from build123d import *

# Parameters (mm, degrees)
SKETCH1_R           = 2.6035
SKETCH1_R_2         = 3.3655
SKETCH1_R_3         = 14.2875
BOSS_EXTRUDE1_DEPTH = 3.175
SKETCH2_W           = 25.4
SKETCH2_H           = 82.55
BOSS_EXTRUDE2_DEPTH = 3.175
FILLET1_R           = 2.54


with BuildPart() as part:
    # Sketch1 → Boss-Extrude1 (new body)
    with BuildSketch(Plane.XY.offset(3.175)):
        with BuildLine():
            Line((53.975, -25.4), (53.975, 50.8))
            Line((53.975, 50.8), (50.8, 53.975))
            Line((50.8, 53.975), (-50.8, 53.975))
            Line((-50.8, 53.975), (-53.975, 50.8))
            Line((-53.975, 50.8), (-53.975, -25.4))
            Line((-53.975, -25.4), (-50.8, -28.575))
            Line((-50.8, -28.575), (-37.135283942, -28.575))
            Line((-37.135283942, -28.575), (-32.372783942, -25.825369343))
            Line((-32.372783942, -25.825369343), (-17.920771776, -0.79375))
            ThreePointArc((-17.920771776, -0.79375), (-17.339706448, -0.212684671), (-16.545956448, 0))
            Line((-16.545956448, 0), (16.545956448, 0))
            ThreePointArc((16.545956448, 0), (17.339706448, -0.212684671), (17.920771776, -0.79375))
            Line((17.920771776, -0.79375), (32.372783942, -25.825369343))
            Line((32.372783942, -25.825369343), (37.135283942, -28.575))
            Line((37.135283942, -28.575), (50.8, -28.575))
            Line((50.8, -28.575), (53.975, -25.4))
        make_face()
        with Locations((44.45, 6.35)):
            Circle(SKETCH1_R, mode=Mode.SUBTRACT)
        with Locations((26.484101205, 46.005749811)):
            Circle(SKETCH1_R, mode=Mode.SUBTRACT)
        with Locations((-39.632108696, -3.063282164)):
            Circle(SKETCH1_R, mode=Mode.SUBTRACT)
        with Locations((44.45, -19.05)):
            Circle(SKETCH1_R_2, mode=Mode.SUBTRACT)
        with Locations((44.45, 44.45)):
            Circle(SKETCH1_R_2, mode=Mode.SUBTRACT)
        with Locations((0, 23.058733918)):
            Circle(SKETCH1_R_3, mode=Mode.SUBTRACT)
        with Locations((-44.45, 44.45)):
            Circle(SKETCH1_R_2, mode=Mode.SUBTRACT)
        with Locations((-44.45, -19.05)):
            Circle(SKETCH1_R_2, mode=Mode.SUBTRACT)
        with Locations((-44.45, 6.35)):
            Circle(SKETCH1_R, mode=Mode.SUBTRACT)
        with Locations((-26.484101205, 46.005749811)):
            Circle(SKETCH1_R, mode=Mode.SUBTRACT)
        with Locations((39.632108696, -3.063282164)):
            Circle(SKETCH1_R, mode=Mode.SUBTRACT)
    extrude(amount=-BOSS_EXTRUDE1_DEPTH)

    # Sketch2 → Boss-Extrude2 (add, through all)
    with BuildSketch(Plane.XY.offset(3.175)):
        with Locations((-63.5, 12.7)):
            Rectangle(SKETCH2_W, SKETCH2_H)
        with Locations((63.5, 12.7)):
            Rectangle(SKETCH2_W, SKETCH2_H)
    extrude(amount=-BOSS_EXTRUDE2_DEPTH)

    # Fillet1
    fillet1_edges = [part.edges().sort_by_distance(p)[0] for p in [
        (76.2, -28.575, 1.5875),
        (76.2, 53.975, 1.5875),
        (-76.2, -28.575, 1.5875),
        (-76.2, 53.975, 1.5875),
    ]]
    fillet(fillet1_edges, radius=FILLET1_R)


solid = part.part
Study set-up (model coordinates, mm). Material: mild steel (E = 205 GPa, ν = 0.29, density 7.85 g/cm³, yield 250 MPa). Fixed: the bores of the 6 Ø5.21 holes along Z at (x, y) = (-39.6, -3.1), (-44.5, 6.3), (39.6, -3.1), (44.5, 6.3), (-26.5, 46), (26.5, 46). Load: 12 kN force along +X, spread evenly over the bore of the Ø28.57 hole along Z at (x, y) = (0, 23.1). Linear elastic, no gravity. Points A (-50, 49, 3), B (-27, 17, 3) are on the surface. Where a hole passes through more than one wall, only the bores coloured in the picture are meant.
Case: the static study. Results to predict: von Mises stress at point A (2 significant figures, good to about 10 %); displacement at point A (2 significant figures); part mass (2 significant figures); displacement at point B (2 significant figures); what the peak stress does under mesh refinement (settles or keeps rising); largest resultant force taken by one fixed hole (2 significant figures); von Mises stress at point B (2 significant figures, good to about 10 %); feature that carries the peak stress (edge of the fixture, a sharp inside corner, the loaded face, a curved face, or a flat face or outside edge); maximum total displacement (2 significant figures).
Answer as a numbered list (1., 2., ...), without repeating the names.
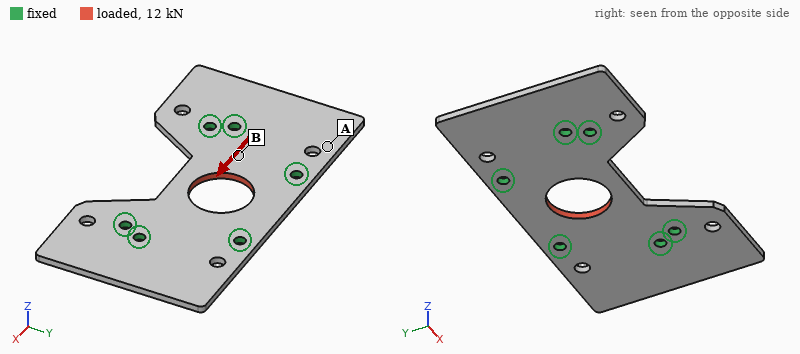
1. 11 MPa
2. 1.8 µm
3. 250 g
4. 4.2 µm
5. keeps rising
6. 3.0 kN
7. 34 MPa
8. edge of the fixture
9. 7.7 µm
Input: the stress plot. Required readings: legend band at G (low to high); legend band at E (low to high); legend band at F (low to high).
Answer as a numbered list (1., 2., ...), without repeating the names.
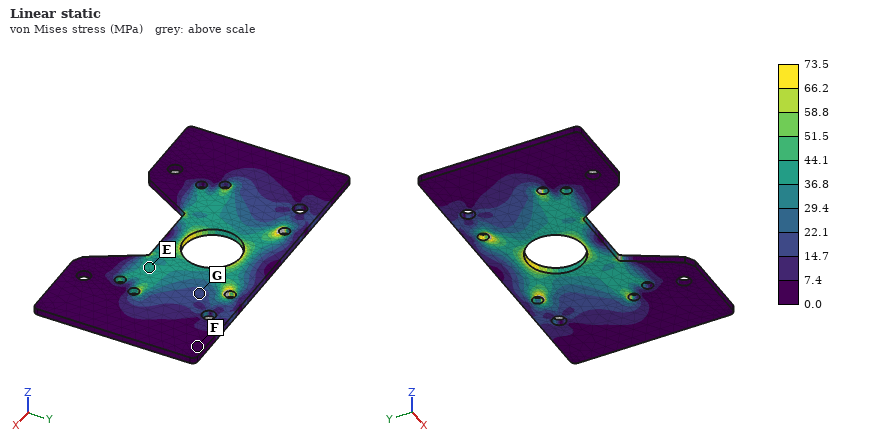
1. 14.7 to 22.1 MPa
2. 36.8 to 44.1 MPa
3. 0.0 to 7.4 MPa
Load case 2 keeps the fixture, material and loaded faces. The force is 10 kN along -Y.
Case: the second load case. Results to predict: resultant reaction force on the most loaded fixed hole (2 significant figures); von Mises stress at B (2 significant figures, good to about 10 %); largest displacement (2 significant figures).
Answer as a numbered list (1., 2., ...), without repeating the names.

1. 3.4 kN
2. 37 MPa
3. 18 µm
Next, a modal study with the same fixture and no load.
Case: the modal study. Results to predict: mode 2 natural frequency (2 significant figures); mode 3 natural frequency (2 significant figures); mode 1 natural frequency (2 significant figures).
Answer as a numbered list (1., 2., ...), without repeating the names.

1. 1700 Hz
2. 2200 Hz
3. 1700 Hz
